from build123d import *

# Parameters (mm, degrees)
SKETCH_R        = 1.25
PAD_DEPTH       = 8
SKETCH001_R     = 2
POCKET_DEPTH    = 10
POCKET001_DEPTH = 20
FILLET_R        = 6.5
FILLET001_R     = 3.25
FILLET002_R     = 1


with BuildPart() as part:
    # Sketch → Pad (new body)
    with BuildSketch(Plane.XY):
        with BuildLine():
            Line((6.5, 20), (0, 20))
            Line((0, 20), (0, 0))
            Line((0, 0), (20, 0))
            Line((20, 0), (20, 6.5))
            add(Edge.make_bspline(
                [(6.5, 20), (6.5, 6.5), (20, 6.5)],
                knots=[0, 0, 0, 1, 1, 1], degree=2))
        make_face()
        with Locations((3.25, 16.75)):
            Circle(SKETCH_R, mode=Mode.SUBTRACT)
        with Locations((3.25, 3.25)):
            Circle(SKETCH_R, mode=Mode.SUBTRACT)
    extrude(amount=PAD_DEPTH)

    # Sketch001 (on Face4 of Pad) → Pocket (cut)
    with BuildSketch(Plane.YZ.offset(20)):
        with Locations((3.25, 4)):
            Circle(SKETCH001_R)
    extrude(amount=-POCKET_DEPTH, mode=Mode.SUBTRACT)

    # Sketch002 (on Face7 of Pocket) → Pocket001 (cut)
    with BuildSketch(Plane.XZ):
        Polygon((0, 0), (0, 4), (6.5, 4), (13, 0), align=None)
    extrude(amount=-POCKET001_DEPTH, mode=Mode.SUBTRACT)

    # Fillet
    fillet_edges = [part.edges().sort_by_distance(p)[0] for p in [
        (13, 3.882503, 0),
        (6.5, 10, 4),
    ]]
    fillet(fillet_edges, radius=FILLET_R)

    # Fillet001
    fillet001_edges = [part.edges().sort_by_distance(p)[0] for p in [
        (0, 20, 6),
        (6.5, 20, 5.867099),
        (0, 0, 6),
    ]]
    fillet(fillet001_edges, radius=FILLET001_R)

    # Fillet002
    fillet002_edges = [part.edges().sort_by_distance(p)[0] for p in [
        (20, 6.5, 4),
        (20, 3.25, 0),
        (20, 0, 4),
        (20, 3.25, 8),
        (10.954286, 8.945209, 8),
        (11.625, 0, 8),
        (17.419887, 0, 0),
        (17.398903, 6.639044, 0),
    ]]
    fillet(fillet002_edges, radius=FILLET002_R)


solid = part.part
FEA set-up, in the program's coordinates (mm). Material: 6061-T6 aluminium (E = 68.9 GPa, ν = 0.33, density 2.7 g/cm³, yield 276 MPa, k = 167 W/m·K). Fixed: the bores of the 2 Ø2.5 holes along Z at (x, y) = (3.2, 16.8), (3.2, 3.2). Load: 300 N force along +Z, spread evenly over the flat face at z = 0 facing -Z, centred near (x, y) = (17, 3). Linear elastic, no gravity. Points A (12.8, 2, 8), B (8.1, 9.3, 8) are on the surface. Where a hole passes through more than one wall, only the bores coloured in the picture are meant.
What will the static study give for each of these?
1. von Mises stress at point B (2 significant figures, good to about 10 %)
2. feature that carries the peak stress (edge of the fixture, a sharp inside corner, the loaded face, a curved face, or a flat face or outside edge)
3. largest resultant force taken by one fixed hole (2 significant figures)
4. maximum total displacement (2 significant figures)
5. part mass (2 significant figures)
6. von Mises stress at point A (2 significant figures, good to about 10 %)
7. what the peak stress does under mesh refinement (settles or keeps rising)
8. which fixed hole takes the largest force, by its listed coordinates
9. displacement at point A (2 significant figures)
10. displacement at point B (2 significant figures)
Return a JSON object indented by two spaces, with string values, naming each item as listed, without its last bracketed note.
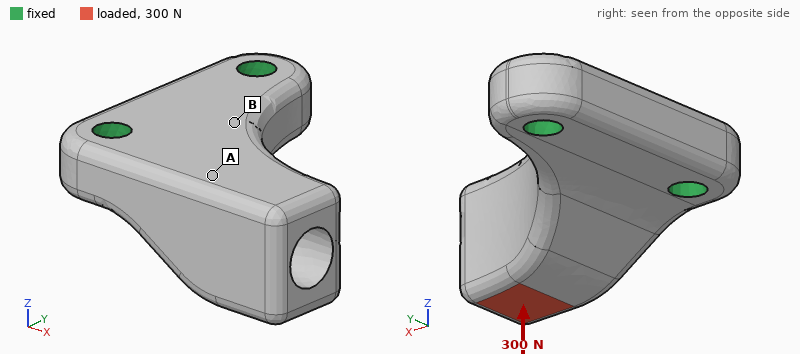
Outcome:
{
  "von Mises stress at point B": "65 MPa",
  "feature that carries the peak stress": "edge of the fixture",
  "largest resultant force taken by one fixed hole": "300 N",
  "maximum total displacement": "79 µm",
  "part mass": "2.9 g",
  "von Mises stress at point A": "23 MPa",
  "what the peak stress does under mesh refinement": "keeps rising",
  "which fixed hole takes the largest force, by its listed coordinates": "(3.2, 3.2)",
  "displacement at point A": "36 µm",
  "displacement at point B": "13 µm"
}
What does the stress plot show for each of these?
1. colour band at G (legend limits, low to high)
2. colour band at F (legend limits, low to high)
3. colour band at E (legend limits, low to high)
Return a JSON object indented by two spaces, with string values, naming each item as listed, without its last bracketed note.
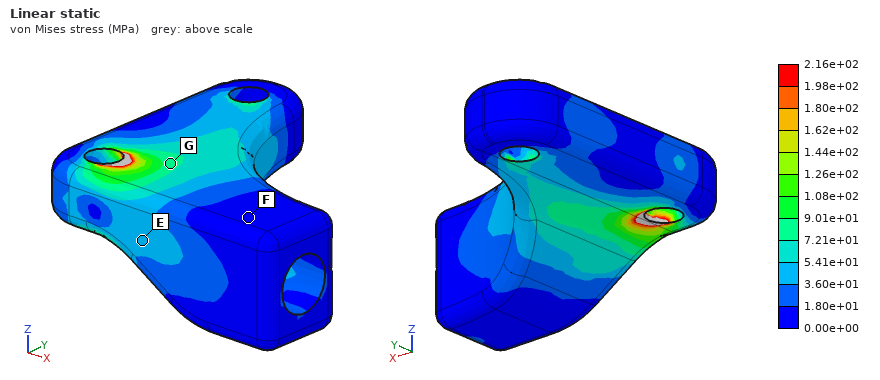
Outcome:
{
  "colour band at G": "7.21e+01 to 9.01e+01 MPa",
  "colour band at F": "0.00e+00 to 1.80e+01 MPa",
  "colour band at E": "3.60e+01 to 5.41e+01 MPa"
}
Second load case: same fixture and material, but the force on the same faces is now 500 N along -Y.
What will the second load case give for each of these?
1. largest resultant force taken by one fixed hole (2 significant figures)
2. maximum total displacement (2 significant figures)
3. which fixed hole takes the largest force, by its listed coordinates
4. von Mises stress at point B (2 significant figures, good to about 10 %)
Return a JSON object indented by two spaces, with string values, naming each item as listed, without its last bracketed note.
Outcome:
{
  "largest resultant force taken by one fixed hole": "630 N",
  "maximum total displacement": "41 µm",
  "which fixed hole takes the largest force, by its listed coordinates": "(3.2, 16.8)",
  "von Mises stress at point B": "22 MPa"
}
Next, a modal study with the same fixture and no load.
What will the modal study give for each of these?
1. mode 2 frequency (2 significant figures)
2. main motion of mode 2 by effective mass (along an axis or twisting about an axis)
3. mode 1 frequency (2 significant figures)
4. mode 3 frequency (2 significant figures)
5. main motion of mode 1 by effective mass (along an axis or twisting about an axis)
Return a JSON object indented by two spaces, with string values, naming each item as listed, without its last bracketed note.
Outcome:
{
  "mode 2 frequency": "26 kHz",
  "main motion of mode 2 by effective mass": "along Y",
  "mode 1 frequency": "12 kHz",
  "mode 3 frequency": "40 kHz",
  "main motion of mode 1 by effective mass": "along Z"
}
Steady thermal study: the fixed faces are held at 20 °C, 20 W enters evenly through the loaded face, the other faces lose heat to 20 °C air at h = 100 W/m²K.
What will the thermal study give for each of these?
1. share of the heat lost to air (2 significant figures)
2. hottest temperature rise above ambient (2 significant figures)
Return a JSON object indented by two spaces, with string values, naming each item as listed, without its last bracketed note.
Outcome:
{
  "share of the heat lost to air": "7.4 %",
  "hottest temperature rise above ambient": "51 K"
}
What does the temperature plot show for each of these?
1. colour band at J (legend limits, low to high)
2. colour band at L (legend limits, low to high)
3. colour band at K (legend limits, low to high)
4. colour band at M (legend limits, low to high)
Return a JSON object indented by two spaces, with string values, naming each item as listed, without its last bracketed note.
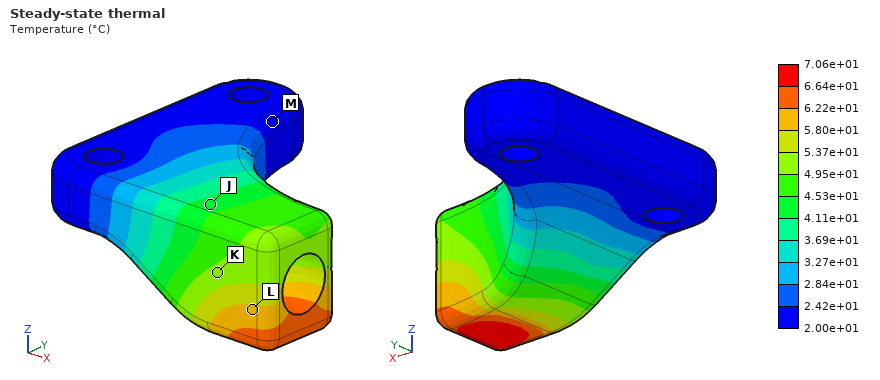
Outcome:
{
  "colour band at J": "4.11e+01 to 4.53e+01 °C",
  "colour band at L": "5.80e+01 to 6.22e+01 °C",
  "colour band at K": "4.95e+01 to 5.37e+01 °C",
  "colour band at M": "2.00e+01 to 2.42e+01 °C"
}
